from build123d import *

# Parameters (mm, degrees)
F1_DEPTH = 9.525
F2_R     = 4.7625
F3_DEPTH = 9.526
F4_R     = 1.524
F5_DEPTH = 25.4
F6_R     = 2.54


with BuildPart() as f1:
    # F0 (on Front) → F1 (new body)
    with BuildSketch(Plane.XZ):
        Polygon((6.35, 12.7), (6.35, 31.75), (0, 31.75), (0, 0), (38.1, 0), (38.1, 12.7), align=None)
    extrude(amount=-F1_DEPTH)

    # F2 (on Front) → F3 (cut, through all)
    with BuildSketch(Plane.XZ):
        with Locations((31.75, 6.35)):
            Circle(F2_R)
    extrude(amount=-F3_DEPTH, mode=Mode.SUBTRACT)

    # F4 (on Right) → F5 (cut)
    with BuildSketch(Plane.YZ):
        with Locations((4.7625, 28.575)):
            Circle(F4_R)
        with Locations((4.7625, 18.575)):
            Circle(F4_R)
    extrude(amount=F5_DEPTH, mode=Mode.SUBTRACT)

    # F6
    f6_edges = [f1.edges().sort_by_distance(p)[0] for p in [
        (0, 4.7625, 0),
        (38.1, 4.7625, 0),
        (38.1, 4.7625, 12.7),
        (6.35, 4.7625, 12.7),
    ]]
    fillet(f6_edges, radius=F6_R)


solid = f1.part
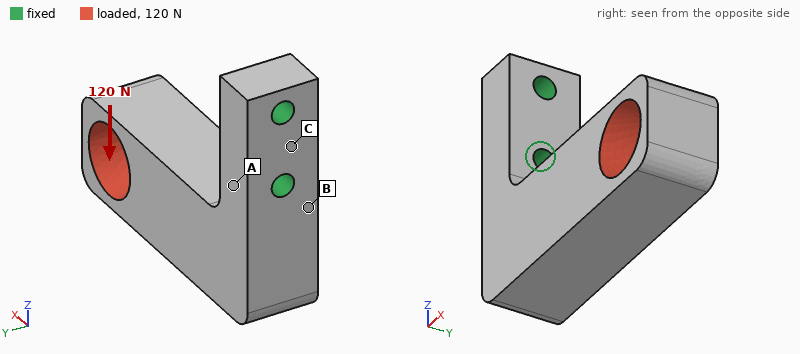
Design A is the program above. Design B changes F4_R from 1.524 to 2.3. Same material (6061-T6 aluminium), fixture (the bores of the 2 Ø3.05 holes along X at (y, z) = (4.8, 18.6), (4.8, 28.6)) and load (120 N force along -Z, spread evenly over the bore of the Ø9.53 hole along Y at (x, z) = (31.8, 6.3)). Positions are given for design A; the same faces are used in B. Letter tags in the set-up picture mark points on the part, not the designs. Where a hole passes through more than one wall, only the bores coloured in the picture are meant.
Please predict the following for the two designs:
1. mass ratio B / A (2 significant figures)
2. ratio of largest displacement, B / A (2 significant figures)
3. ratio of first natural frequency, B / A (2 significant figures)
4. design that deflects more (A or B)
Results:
0.98
0.88
1.1
A
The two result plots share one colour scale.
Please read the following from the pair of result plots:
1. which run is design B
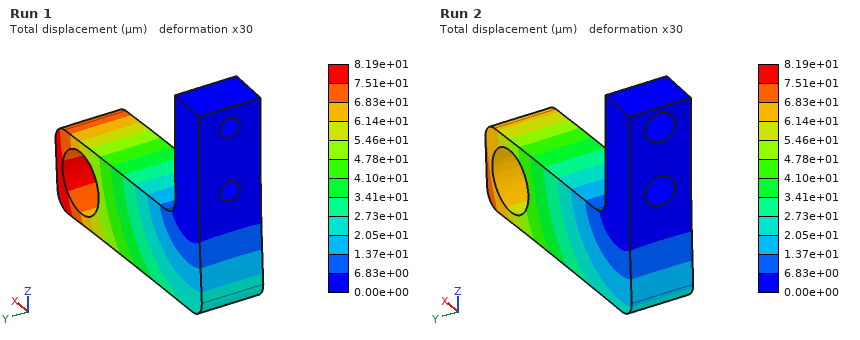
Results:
Run 2
